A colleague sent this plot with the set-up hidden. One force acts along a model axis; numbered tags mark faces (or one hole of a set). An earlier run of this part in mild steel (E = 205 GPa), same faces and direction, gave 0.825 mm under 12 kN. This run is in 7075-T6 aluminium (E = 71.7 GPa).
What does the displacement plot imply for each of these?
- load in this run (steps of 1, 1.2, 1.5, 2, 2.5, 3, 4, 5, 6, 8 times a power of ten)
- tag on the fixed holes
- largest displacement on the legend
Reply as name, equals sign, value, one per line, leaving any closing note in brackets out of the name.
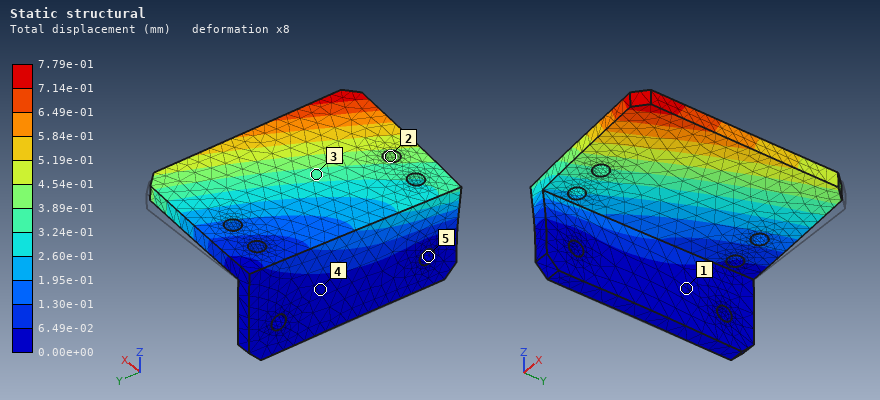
load in this run = 4 kN
tag on the fixed holes = 5
largest displacement on the legend = 7.79e-01 mm
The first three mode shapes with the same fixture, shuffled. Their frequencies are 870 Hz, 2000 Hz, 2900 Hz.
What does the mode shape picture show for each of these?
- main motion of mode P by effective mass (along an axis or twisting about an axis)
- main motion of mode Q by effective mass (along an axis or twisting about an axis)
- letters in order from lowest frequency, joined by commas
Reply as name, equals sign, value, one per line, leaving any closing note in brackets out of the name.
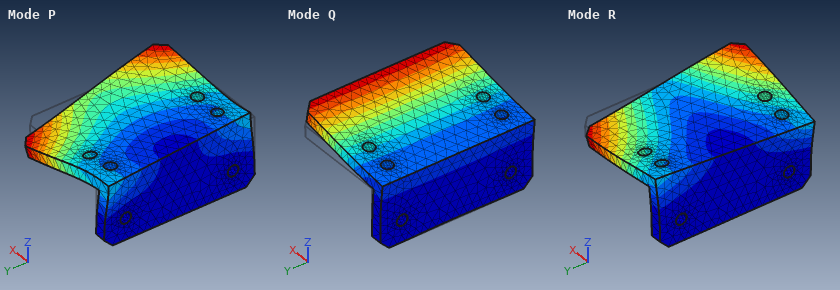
main motion of mode P by effective mass = along Y
main motion of mode Q by effective mass = along Z
letters in order from lowest frequency, joined by commas = Q, R, P
